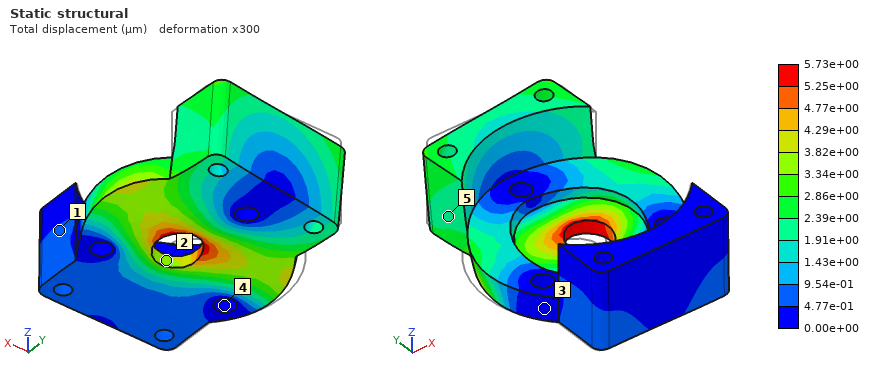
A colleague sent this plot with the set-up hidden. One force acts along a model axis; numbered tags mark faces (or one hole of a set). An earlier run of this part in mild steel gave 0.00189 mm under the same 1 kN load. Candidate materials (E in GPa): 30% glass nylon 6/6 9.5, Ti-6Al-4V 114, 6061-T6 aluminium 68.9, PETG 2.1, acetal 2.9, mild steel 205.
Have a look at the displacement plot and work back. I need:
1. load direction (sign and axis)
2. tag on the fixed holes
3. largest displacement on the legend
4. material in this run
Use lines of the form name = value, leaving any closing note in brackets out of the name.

load direction = +X
tag on the fixed holes = 4
largest displacement on the legend = 5.73e+00 µm
material in this run = 6061-T6 aluminium
